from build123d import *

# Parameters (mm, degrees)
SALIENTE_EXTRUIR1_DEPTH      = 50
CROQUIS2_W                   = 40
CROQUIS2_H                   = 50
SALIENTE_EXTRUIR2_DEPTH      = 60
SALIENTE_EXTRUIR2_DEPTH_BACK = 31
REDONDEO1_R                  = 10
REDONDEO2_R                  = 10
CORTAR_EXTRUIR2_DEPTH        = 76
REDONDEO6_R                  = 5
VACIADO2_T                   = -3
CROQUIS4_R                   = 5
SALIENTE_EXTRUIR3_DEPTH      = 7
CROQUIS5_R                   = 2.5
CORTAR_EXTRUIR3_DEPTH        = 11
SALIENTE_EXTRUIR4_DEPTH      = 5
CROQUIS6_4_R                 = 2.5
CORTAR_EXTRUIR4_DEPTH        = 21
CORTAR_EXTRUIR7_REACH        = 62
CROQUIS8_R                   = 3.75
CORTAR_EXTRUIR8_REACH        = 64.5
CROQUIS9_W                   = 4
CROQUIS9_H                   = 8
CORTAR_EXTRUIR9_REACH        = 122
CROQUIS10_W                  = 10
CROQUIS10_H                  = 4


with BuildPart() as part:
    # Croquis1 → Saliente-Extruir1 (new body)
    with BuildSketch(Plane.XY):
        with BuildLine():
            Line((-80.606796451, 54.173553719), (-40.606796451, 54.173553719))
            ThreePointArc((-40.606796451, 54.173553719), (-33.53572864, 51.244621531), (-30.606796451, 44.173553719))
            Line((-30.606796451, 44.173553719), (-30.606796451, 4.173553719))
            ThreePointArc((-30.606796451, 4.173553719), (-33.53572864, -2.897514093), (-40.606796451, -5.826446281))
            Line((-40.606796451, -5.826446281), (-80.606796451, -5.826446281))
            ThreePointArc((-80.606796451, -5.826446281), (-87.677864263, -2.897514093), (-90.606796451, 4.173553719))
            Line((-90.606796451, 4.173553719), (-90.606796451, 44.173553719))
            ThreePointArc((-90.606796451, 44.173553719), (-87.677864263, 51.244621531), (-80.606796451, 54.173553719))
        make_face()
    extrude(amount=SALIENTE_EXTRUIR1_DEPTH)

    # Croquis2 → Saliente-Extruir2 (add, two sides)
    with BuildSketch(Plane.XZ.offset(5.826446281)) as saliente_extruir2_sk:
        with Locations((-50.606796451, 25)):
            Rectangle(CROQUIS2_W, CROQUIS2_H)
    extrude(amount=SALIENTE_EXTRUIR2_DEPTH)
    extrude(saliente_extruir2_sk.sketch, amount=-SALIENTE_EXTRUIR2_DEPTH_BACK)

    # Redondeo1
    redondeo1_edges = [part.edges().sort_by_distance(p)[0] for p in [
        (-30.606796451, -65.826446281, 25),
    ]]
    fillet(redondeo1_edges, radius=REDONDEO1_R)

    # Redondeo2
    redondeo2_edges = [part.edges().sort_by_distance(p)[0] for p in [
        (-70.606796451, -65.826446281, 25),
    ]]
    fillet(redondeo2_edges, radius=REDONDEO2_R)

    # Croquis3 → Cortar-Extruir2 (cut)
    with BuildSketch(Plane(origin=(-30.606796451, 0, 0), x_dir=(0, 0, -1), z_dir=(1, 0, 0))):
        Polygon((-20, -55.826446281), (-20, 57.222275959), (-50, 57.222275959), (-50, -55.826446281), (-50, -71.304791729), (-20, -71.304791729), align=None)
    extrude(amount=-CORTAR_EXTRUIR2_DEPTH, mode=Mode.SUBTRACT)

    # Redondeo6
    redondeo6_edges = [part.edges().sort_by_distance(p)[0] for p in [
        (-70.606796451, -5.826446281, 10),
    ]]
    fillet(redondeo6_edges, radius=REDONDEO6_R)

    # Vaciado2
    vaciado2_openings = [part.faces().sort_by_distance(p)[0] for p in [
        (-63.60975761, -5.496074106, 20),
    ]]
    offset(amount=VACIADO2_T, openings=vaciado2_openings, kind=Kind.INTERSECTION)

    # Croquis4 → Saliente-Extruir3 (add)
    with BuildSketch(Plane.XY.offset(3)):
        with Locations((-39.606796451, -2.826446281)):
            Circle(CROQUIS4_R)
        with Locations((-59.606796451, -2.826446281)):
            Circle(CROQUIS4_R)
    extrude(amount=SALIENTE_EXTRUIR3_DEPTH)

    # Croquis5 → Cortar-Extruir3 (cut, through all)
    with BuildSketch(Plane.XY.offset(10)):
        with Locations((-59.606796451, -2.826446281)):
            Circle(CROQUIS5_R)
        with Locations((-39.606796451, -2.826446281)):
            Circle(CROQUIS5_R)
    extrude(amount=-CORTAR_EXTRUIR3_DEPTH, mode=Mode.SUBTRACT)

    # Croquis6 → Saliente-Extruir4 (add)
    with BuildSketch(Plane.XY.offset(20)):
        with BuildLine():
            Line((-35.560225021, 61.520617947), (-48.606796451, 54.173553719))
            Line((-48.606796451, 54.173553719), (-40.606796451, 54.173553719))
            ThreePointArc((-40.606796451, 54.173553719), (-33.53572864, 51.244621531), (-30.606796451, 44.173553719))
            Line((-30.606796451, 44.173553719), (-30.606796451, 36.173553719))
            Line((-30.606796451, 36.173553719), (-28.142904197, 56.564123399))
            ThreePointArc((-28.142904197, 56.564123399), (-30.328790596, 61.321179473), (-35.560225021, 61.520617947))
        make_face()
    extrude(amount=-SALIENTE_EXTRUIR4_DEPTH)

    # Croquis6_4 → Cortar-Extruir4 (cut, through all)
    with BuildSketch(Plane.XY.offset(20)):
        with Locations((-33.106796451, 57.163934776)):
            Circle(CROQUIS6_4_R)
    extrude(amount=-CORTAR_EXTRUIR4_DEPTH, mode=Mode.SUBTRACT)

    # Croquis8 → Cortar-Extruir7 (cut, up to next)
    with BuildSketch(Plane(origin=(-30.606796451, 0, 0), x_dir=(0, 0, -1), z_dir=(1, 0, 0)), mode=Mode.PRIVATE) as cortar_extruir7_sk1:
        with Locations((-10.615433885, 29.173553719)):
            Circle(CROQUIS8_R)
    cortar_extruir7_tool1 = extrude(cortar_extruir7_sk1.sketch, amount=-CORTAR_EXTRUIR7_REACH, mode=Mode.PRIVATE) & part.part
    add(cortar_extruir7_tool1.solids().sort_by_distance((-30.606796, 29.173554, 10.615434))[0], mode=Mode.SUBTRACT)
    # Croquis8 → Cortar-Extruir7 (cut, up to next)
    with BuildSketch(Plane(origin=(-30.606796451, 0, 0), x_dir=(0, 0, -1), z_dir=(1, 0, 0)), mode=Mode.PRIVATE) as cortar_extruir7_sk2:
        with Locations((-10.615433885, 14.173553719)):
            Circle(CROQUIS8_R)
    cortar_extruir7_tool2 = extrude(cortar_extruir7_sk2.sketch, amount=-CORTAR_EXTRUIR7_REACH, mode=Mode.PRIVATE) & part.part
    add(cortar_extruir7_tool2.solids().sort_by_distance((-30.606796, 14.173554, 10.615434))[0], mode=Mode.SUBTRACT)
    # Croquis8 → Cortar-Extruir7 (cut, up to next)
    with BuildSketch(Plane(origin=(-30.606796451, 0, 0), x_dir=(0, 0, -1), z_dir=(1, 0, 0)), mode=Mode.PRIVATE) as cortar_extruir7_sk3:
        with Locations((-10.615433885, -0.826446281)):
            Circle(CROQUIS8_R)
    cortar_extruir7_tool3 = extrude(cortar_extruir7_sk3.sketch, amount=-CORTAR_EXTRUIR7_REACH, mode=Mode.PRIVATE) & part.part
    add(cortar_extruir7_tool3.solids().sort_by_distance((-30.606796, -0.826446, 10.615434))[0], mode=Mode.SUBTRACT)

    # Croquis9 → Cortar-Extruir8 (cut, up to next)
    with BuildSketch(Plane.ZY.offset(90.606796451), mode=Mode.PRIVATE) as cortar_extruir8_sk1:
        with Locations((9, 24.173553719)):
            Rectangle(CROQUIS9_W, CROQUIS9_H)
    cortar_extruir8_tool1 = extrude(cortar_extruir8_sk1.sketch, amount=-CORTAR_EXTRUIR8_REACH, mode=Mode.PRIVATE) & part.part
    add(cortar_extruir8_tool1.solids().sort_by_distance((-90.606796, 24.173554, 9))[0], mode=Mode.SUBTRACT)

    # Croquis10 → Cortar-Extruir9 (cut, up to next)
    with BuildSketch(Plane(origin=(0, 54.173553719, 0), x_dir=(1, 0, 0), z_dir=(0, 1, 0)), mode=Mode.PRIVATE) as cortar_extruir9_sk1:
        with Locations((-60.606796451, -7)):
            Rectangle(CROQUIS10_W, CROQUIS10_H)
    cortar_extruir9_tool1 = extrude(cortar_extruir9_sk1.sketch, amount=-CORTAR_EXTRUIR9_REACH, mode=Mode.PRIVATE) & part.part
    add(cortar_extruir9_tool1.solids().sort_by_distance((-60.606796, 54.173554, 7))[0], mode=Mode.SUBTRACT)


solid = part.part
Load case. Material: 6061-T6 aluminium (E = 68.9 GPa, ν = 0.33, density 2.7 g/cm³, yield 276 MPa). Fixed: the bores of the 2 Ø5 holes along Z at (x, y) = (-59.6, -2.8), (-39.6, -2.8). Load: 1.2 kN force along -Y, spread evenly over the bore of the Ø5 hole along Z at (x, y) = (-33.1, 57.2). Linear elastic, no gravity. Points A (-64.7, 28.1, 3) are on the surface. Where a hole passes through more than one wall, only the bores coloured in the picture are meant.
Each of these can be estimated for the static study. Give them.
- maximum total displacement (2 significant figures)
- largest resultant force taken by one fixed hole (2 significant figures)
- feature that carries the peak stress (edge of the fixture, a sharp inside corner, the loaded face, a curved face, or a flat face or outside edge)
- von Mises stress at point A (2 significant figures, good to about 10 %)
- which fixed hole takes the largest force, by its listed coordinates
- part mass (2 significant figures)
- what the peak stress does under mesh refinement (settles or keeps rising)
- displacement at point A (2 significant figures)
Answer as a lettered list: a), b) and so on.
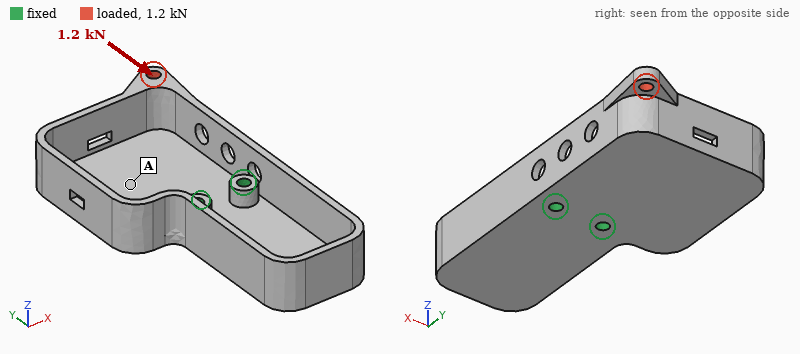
a) 0.58 mm
b) 1.4 kN
c) a sharp inside corner
d) 15 MPa
e) (-39.6, -2.8)
f) 95 g
g) keeps rising
h) 0.14 mm
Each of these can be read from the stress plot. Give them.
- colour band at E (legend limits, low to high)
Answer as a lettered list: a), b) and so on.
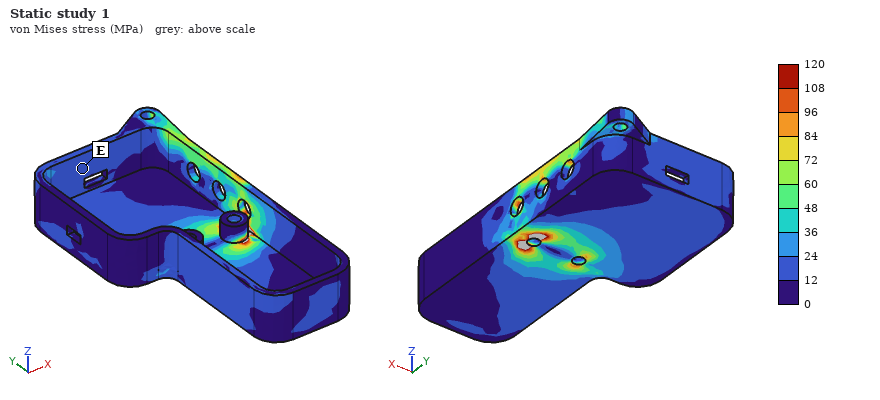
a) 12 to 24 MPa
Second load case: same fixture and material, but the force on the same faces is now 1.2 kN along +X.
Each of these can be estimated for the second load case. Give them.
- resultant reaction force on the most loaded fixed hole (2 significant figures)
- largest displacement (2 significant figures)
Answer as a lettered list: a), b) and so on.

a) 3.0 kN
b) 0.87 mm
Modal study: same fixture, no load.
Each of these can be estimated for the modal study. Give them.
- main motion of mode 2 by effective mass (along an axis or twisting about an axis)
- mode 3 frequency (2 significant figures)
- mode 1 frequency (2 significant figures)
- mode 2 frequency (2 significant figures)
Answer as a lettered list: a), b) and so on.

a) along Z
b) 1500 Hz
c) 760 Hz
d) 1200 Hz
